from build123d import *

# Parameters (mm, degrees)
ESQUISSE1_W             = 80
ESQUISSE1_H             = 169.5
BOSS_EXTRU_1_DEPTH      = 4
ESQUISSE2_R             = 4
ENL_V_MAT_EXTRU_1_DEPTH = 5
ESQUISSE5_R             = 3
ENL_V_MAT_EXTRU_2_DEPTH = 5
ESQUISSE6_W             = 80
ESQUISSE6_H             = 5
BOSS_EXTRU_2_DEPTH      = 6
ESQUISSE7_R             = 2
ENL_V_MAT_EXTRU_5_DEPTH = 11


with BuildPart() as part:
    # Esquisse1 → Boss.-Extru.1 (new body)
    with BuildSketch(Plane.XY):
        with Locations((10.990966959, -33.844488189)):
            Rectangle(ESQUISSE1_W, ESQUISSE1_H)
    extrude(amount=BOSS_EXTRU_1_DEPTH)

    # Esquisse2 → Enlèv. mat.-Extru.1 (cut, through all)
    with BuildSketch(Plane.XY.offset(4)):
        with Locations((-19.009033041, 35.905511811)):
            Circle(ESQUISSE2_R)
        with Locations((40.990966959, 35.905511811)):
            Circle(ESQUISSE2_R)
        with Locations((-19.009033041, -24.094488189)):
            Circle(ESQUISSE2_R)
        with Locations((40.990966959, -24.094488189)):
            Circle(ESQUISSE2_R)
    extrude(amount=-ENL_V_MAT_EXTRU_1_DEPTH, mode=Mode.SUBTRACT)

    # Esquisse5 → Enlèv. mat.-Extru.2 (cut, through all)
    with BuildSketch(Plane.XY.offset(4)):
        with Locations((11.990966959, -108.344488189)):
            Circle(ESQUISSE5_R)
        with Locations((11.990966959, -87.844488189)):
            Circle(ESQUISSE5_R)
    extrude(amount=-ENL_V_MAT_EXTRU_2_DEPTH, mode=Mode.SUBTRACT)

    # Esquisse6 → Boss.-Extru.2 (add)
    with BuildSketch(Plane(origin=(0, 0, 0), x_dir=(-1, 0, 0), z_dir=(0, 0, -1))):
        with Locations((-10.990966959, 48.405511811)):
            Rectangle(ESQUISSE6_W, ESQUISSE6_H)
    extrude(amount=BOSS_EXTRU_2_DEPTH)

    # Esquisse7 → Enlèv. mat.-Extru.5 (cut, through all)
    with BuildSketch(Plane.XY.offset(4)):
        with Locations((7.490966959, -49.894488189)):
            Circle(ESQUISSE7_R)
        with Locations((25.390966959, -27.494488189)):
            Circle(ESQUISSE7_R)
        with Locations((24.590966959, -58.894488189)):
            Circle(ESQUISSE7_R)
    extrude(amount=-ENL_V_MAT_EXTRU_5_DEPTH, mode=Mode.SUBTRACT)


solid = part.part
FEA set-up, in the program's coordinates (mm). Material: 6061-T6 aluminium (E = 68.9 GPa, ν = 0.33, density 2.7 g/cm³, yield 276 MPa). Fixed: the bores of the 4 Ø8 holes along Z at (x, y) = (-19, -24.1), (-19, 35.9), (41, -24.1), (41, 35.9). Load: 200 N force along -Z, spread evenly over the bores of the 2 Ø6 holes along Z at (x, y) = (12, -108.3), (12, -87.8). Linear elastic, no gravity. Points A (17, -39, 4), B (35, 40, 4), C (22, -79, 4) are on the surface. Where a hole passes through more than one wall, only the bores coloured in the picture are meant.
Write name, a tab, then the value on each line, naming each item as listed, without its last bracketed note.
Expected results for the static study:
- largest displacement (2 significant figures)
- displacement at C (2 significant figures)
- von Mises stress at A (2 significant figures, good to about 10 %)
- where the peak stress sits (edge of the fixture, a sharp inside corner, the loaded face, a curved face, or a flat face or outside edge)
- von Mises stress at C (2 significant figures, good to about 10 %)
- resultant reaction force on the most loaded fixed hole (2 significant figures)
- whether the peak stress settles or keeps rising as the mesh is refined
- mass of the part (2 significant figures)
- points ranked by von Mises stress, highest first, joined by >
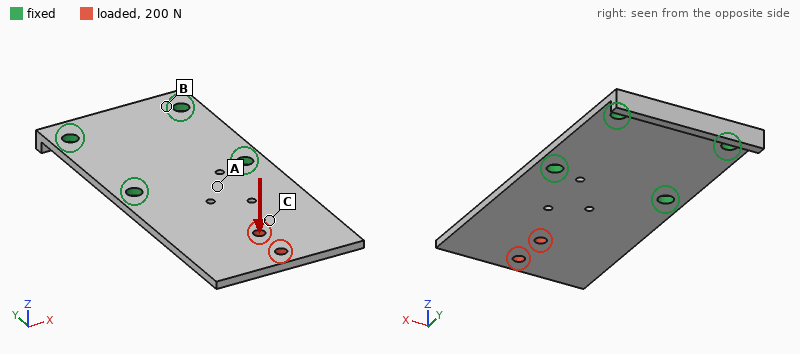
largest displacement	1.3 mm
displacement at C	0.60 mm
von Mises stress at A	45 MPa
where the peak stress sits	edge of the fixture
von Mises stress at C	20 MPa
resultant reaction force on the most loaded fixed hole	120 N
whether the peak stress settles or keeps rising as the mesh is refined	keeps rising
mass of the part	150 g
points ranked by von Mises stress, highest first, joined by >	A > C > B
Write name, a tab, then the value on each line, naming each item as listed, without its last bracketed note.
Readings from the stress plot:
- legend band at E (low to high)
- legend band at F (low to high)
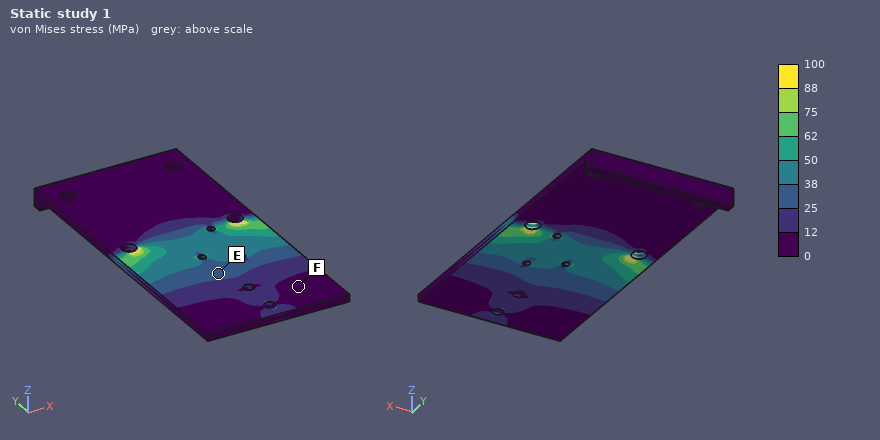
legend band at E	25 to 38 MPa
legend band at F	0 to 12 MPa
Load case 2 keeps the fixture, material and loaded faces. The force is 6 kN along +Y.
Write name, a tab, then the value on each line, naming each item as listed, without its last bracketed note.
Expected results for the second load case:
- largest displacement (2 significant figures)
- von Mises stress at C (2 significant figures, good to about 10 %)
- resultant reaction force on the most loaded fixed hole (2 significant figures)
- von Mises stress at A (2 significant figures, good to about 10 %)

largest displacement	37 µm
von Mises stress at C	30 MPa
resultant reaction force on the most loaded fixed hole	2.7 kN
von Mises stress at A	14 MPa
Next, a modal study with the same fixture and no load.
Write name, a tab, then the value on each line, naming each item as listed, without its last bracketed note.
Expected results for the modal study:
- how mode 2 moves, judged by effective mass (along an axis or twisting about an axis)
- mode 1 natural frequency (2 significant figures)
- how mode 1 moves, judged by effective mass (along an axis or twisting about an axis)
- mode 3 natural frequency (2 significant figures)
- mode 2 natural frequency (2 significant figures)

how mode 2 moves, judged by effective mass	twisting about Y
mode 1 natural frequency	370 Hz
how mode 1 moves, judged by effective mass	along Z
mode 3 natural frequency	2300 Hz
mode 2 natural frequency	1000 Hz
